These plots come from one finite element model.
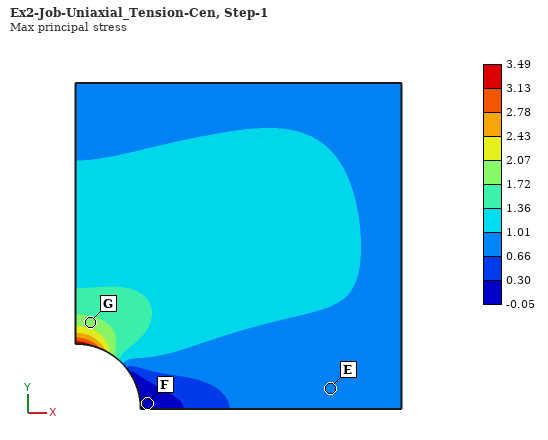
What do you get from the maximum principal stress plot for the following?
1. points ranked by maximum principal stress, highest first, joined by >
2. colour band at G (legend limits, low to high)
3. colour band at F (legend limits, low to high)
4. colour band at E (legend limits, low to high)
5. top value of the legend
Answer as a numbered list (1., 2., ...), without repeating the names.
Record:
1. G > E > F
2. 1.72 to 2.07
3. -0.05 to 0.30
4. 0.66 to 1.01
5. 3.49
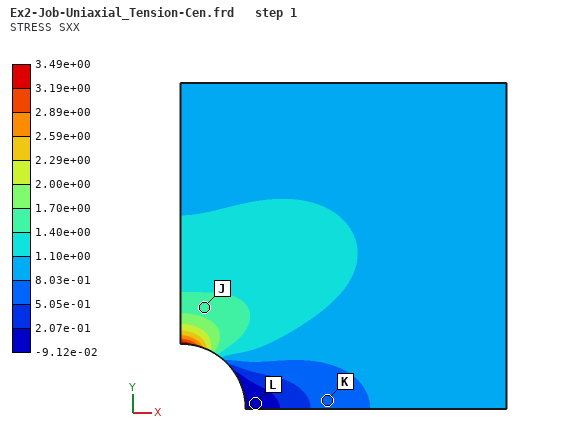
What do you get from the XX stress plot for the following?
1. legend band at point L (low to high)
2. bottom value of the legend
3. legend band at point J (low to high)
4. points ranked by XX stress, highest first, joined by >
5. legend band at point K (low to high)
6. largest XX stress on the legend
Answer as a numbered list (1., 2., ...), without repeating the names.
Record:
1. -9.12e-02 to 2.07e-01
2. -9.12e-02
3. 1.40e+00 to 1.70e+00
4. J > K > L
5. 5.05e-01 to 8.03e-01
6. 3.49e+00
